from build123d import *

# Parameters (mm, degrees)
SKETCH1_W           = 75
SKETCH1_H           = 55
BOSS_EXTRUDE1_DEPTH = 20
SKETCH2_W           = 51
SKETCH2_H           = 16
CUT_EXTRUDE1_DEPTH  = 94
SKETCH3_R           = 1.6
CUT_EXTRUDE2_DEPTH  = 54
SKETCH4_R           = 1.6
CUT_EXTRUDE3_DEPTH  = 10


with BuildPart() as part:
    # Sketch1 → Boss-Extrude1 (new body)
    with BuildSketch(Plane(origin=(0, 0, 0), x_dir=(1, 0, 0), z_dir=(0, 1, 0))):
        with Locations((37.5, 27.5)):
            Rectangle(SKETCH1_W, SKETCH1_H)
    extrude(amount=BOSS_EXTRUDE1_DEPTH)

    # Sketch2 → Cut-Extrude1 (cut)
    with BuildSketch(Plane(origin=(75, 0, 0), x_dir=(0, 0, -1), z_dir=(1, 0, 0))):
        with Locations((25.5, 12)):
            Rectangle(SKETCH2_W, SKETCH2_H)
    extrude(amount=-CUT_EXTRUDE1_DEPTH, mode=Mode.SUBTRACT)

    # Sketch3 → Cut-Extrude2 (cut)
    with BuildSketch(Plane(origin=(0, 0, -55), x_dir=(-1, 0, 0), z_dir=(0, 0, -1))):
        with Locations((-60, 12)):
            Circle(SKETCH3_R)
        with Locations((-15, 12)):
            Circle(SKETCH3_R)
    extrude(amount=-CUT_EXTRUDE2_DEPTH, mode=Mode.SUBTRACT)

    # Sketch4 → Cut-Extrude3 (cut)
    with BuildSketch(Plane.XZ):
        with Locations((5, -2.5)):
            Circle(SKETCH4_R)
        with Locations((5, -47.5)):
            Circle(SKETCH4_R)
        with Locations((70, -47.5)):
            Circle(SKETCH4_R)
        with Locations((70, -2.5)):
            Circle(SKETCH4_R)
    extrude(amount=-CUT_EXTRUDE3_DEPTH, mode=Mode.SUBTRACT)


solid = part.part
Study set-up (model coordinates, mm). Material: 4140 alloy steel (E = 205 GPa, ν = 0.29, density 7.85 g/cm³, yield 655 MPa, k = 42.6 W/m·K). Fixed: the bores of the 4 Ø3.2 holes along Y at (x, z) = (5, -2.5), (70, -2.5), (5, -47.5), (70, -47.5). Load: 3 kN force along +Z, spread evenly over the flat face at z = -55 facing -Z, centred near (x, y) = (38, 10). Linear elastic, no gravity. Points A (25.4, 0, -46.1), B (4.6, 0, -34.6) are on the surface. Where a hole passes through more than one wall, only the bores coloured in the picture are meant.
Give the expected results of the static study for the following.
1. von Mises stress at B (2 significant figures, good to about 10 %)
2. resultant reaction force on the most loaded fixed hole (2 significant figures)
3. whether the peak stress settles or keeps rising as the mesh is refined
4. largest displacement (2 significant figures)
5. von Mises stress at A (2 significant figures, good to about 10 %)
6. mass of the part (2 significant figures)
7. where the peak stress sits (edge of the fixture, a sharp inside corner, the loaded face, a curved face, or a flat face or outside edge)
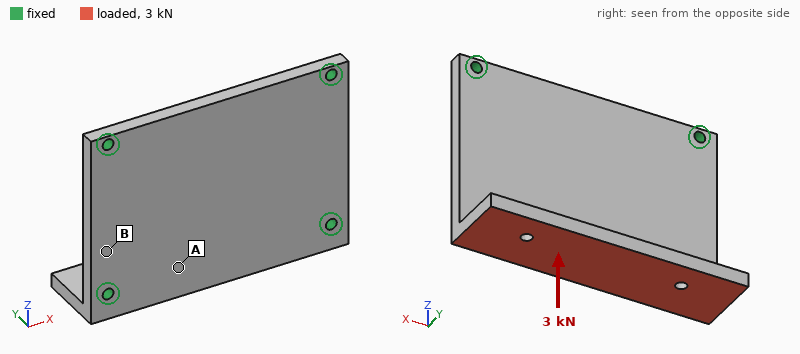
20 MPa
1.1 kN
keeps rising
75 µm
57 MPa
170 g
edge of the fixture
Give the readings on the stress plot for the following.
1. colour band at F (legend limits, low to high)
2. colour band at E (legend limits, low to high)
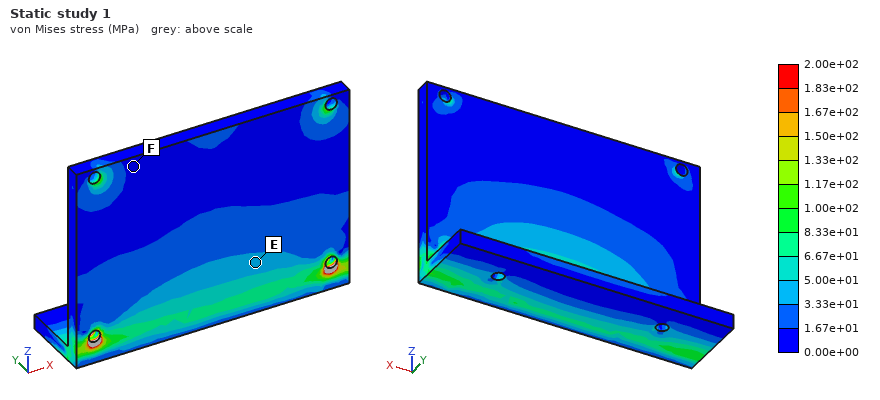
0.00e+00 to 1.67e+01 MPa
3.33e+01 to 5.00e+01 MPa
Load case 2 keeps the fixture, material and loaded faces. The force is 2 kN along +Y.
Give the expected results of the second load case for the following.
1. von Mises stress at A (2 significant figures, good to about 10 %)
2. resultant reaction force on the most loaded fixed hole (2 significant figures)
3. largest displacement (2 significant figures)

23 MPa
1.2 kN
30 µm
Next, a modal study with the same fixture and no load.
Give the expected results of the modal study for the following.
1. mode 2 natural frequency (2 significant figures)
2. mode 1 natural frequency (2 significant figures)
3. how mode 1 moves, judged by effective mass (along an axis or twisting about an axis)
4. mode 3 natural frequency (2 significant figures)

6000 Hz
4200 Hz
along Y
8200 Hz
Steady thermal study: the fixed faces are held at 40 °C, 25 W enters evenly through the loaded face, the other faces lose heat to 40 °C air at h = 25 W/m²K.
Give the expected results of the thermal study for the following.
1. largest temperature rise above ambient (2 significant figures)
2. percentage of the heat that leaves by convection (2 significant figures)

45 K
16 %
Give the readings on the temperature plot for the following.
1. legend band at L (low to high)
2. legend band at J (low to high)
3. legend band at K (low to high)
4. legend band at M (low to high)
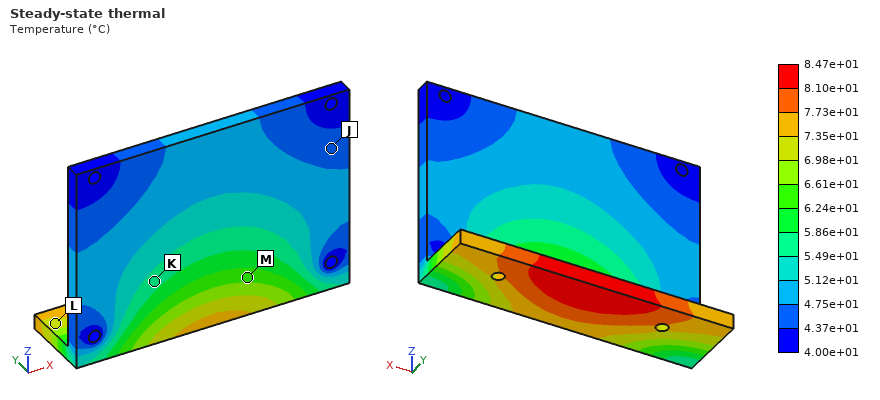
6.98e+01 to 7.35e+01 °C
4.37e+01 to 4.75e+01 °C
5.49e+01 to 5.86e+01 °C
6.24e+01 to 6.61e+01 °C
